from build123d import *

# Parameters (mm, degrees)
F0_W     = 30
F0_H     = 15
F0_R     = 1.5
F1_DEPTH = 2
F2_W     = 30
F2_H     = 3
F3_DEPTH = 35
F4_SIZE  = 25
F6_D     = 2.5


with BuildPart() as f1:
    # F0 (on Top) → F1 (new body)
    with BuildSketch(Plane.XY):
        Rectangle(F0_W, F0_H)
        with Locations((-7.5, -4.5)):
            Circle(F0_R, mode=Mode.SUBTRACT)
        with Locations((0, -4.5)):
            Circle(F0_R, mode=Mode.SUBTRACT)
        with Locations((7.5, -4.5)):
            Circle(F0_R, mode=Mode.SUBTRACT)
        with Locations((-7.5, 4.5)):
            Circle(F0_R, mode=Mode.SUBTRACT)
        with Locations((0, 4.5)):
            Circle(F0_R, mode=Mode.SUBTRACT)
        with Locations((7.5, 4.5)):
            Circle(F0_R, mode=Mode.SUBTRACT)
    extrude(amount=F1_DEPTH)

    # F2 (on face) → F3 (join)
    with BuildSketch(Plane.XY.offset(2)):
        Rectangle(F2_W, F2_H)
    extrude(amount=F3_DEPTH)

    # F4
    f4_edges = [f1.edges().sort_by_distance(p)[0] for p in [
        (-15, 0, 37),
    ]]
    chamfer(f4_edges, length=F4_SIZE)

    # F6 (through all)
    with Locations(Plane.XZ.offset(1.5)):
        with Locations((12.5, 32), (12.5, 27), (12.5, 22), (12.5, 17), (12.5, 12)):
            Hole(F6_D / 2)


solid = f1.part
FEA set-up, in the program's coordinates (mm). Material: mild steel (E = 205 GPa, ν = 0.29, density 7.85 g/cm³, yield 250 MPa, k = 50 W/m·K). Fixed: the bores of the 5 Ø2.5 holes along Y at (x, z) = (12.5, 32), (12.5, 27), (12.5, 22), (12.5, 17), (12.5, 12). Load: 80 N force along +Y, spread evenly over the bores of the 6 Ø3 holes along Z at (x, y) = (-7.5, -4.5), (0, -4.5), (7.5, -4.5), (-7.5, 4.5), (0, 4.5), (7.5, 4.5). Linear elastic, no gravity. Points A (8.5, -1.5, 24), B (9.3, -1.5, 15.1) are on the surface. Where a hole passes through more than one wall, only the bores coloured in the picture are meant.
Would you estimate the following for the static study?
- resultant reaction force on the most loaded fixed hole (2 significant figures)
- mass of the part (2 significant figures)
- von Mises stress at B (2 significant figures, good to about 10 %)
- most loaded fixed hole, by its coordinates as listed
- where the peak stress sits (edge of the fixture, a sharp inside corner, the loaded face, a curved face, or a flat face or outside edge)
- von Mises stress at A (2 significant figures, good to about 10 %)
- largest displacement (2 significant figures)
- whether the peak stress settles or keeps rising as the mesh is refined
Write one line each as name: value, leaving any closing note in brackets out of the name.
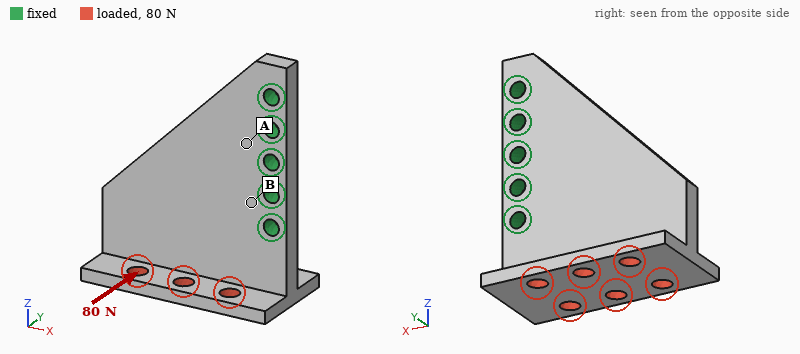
resultant reaction force on the most loaded fixed hole: 110 N
mass of the part: 23 g
von Mises stress at B: 28 MPa
most loaded fixed hole, by its coordinates as listed: (12.5, 12)
where the peak stress sits: edge of the fixture
von Mises stress at A: 9.0 MPa
largest displacement: 28 µm
whether the peak stress settles or keeps rising as the mesh is refined: keeps rising
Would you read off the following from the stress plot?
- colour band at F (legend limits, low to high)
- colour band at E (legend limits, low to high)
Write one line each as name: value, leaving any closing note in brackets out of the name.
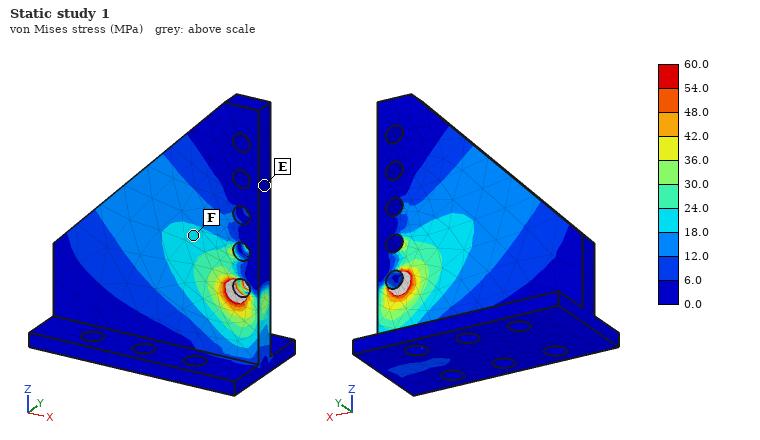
colour band at F: 18.0 to 24.0 MPa
colour band at E: 0.0 to 6.0 MPa
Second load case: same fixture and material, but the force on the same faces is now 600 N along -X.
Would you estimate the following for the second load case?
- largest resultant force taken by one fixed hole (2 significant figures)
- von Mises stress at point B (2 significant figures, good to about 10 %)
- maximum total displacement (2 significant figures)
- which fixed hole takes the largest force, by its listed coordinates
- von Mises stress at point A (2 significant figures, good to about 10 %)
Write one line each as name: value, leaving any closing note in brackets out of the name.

largest resultant force taken by one fixed hole: 860 N
von Mises stress at point B: 16 MPa
maximum total displacement: 7.4 µm
which fixed hole takes the largest force, by its listed coordinates: (12.5, 12)
von Mises stress at point A: 12 MPa
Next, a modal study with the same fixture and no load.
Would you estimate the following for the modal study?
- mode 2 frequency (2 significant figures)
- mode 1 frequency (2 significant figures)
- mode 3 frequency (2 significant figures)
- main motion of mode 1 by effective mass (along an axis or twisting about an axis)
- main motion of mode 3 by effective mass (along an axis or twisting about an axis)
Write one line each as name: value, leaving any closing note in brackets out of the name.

mode 2 frequency: 7800 Hz
mode 1 frequency: 3000 Hz
mode 3 frequency: 13 kHz
main motion of mode 1 by effective mass: along Y
main motion of mode 3 by effective mass: along Y
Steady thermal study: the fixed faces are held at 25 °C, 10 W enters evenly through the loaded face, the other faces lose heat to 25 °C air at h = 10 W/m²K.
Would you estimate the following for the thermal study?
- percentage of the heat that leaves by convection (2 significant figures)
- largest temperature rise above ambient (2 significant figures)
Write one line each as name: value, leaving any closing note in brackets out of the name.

percentage of the heat that leaves by convection: 7.4 %
largest temperature rise above ambient: 57 K
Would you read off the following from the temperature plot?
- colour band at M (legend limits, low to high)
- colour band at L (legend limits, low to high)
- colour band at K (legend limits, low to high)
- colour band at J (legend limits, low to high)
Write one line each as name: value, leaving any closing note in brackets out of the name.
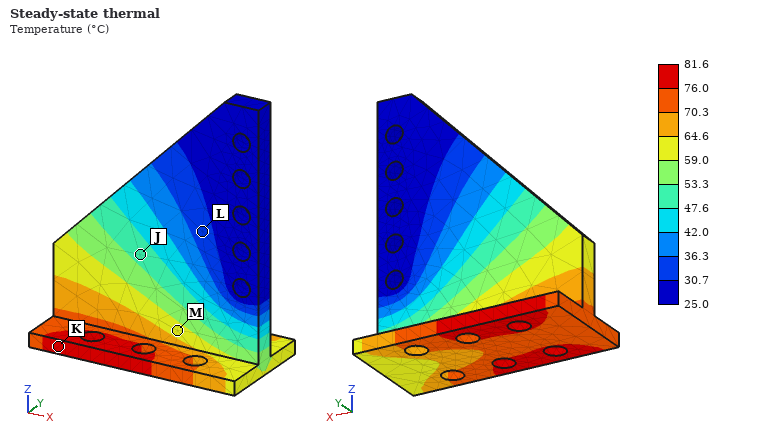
colour band at M: 59.0 to 64.6 °C
colour band at L: 30.7 to 36.3 °C
colour band at K: 76.0 to 81.6 °C
colour band at J: 47.6 to 53.3 °C
